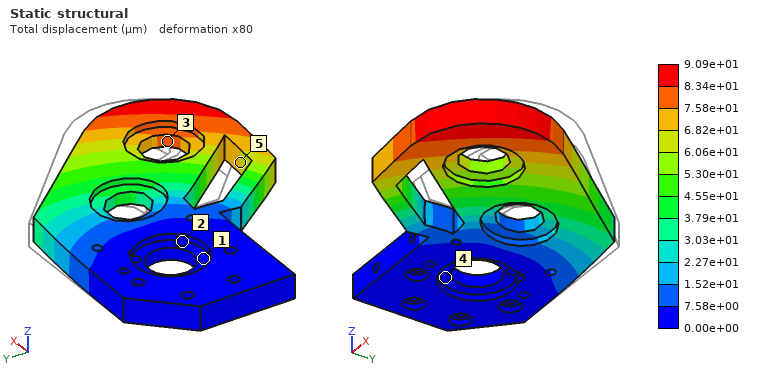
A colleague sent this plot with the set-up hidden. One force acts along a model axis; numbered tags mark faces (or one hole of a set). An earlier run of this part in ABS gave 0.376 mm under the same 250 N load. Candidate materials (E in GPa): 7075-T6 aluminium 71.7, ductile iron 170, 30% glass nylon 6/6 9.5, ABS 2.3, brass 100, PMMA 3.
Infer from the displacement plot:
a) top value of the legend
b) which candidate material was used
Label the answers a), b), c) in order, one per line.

a) 9.09e+01 µm
b) 30% glass nylon 6/6
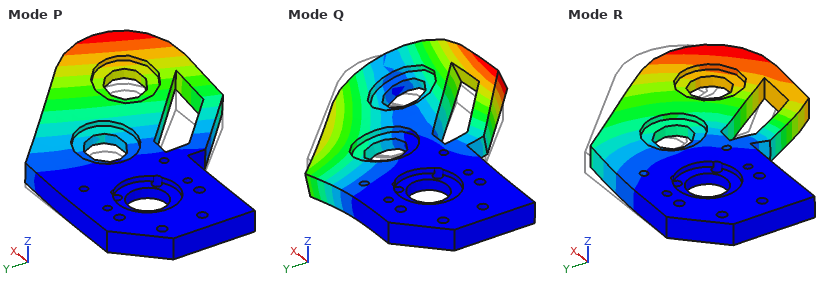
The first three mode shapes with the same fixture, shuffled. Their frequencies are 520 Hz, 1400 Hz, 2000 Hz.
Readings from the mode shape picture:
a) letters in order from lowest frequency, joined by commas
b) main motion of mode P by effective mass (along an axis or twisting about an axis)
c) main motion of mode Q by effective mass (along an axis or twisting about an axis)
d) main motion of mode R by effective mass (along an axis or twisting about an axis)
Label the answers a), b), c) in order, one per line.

a) P, Q, R
b) along Z
c) twisting about X
d) along Y
